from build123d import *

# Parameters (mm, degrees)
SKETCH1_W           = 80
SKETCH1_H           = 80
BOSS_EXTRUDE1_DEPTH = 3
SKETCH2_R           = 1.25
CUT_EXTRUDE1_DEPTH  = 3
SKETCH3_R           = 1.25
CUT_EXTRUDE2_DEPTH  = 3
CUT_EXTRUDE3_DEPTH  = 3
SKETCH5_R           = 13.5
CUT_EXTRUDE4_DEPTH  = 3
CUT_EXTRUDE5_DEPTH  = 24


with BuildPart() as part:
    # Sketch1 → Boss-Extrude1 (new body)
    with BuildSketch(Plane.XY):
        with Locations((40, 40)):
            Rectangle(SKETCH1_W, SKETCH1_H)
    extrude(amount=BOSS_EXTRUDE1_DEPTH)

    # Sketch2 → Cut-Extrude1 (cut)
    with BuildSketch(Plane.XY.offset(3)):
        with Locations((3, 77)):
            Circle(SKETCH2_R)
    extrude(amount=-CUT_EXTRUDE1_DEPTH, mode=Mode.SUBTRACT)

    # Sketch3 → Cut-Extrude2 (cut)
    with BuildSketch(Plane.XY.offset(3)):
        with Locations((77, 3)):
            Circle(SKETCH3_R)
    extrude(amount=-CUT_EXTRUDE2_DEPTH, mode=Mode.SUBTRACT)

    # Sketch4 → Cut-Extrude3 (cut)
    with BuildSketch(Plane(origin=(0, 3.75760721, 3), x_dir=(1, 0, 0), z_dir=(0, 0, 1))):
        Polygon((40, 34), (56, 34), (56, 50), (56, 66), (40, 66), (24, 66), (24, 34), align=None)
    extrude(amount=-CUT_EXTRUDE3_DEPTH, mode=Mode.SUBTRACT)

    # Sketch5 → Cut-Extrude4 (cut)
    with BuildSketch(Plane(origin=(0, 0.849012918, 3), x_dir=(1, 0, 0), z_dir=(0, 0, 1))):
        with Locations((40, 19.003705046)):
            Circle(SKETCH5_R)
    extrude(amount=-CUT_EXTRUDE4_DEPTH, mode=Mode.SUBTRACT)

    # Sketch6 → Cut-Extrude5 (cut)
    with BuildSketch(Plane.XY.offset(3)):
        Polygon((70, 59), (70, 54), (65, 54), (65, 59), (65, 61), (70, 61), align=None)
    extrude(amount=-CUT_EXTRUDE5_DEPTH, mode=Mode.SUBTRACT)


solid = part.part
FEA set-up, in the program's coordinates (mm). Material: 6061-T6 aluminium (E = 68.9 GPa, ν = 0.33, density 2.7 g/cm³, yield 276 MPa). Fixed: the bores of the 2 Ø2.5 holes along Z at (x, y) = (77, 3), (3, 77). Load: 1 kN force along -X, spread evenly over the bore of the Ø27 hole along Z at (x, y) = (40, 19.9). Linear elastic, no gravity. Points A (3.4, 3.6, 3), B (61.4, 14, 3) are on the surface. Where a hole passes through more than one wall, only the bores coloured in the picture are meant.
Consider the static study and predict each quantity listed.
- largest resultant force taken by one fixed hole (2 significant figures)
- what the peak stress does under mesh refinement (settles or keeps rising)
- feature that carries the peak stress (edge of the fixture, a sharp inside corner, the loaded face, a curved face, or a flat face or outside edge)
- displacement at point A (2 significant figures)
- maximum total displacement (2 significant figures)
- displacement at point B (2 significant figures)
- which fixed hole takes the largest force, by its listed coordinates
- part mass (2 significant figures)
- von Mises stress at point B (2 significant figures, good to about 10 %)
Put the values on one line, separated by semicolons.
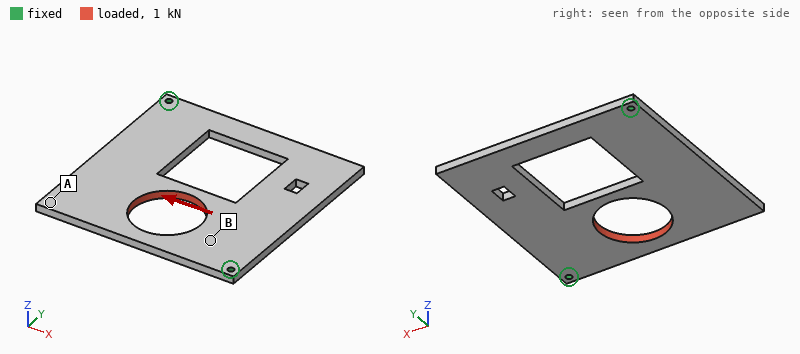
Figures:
780 N; keeps rising; edge of the fixture; 17 µm; 18 µm; 11 µm; (77, 3); 39 g; 7.7 MPa
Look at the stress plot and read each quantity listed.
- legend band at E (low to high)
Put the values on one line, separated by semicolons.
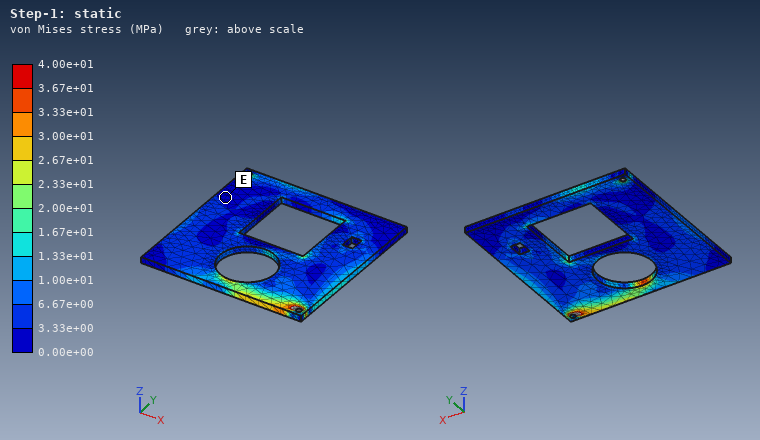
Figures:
0.00e+00 to 3.33e+00 MPa
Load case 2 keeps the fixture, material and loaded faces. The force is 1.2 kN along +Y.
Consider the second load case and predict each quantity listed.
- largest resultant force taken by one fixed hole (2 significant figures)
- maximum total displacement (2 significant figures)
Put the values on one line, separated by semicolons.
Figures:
600 N; 22 µm
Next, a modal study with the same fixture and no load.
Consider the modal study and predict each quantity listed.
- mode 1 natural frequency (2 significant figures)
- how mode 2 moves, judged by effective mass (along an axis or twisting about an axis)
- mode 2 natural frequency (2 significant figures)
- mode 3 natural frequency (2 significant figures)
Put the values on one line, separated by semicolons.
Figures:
560 Hz; along Z; 720 Hz; 2000 Hz
